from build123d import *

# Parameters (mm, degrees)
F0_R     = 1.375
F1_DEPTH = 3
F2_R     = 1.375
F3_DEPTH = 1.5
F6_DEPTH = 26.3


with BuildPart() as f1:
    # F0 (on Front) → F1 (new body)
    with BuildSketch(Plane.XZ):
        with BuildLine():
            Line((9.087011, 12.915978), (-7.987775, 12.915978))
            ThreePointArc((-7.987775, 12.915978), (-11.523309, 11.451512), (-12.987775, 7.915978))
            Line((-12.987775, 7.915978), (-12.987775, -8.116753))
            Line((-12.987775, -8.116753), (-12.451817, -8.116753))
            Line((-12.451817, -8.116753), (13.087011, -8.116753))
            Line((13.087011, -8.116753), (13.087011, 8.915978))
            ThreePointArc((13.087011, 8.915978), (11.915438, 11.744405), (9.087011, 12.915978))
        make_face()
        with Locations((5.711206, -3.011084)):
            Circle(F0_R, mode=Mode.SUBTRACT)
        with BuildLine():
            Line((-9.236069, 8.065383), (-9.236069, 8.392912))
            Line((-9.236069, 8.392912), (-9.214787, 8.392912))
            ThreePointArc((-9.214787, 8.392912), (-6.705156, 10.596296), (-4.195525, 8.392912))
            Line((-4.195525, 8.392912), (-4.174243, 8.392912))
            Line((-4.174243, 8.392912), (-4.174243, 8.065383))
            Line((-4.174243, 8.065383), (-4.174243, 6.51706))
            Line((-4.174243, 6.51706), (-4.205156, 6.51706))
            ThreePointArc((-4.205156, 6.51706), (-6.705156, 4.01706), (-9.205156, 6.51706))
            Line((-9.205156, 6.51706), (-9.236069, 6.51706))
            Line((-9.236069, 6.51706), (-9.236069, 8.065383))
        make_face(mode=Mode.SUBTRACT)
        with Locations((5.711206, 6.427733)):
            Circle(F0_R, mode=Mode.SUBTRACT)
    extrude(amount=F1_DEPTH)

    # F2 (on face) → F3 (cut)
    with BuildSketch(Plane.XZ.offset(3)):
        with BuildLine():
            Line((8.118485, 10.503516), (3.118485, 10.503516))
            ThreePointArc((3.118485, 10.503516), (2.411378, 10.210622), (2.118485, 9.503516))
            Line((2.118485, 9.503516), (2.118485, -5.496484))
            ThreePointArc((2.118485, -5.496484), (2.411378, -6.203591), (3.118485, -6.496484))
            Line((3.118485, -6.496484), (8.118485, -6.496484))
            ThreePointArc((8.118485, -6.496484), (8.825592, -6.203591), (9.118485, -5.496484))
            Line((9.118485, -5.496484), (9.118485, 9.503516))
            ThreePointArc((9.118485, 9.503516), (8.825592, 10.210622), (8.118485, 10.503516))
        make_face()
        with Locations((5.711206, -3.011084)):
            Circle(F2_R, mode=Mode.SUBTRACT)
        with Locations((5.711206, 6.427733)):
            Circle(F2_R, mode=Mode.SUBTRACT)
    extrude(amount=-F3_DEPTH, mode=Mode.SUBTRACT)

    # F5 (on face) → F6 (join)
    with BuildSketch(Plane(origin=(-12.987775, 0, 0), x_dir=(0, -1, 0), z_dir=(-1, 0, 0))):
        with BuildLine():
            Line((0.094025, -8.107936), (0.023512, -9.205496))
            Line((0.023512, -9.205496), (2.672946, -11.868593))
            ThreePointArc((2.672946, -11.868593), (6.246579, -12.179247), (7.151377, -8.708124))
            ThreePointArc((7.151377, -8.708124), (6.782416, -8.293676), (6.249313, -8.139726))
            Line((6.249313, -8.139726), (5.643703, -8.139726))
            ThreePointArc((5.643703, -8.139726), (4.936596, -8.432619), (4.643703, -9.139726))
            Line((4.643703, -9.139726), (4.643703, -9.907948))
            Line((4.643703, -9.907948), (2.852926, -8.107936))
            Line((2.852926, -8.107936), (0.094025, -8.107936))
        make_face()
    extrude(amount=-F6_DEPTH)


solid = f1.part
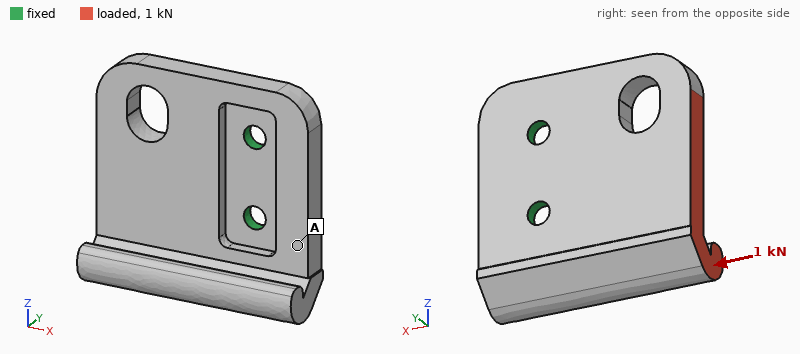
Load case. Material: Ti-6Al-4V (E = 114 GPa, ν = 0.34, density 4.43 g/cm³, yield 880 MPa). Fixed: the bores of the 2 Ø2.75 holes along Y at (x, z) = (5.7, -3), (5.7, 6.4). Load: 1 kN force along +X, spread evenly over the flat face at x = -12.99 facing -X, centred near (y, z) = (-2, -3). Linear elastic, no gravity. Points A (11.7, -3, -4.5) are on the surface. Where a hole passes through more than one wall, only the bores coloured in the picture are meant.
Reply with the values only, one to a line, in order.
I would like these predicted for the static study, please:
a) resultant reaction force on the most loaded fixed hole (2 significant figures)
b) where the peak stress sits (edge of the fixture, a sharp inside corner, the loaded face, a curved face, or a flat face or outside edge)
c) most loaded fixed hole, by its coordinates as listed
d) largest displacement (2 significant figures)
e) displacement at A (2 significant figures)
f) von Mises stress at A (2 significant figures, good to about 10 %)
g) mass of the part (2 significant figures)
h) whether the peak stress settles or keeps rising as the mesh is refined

950 N
edge of the fixture
(5.7, -3)
73 µm
16 µm
30 MPa
8.7 g
keeps rising
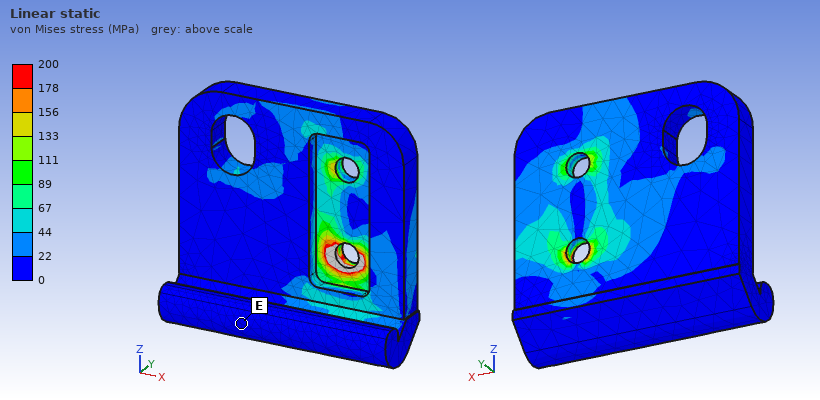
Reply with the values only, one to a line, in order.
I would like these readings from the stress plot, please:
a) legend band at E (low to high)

0 to 22 MPa
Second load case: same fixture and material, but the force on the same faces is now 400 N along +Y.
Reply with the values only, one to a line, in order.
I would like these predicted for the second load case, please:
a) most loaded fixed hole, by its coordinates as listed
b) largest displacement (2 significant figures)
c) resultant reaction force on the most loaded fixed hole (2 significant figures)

(5.7, -3)
0.33 mm
390 N
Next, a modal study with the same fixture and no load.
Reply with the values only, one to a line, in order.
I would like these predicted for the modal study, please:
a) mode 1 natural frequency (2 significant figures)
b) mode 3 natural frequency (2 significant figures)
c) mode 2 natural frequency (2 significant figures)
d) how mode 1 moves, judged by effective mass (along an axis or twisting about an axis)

4000 Hz
13 kHz
8100 Hz
along Y
